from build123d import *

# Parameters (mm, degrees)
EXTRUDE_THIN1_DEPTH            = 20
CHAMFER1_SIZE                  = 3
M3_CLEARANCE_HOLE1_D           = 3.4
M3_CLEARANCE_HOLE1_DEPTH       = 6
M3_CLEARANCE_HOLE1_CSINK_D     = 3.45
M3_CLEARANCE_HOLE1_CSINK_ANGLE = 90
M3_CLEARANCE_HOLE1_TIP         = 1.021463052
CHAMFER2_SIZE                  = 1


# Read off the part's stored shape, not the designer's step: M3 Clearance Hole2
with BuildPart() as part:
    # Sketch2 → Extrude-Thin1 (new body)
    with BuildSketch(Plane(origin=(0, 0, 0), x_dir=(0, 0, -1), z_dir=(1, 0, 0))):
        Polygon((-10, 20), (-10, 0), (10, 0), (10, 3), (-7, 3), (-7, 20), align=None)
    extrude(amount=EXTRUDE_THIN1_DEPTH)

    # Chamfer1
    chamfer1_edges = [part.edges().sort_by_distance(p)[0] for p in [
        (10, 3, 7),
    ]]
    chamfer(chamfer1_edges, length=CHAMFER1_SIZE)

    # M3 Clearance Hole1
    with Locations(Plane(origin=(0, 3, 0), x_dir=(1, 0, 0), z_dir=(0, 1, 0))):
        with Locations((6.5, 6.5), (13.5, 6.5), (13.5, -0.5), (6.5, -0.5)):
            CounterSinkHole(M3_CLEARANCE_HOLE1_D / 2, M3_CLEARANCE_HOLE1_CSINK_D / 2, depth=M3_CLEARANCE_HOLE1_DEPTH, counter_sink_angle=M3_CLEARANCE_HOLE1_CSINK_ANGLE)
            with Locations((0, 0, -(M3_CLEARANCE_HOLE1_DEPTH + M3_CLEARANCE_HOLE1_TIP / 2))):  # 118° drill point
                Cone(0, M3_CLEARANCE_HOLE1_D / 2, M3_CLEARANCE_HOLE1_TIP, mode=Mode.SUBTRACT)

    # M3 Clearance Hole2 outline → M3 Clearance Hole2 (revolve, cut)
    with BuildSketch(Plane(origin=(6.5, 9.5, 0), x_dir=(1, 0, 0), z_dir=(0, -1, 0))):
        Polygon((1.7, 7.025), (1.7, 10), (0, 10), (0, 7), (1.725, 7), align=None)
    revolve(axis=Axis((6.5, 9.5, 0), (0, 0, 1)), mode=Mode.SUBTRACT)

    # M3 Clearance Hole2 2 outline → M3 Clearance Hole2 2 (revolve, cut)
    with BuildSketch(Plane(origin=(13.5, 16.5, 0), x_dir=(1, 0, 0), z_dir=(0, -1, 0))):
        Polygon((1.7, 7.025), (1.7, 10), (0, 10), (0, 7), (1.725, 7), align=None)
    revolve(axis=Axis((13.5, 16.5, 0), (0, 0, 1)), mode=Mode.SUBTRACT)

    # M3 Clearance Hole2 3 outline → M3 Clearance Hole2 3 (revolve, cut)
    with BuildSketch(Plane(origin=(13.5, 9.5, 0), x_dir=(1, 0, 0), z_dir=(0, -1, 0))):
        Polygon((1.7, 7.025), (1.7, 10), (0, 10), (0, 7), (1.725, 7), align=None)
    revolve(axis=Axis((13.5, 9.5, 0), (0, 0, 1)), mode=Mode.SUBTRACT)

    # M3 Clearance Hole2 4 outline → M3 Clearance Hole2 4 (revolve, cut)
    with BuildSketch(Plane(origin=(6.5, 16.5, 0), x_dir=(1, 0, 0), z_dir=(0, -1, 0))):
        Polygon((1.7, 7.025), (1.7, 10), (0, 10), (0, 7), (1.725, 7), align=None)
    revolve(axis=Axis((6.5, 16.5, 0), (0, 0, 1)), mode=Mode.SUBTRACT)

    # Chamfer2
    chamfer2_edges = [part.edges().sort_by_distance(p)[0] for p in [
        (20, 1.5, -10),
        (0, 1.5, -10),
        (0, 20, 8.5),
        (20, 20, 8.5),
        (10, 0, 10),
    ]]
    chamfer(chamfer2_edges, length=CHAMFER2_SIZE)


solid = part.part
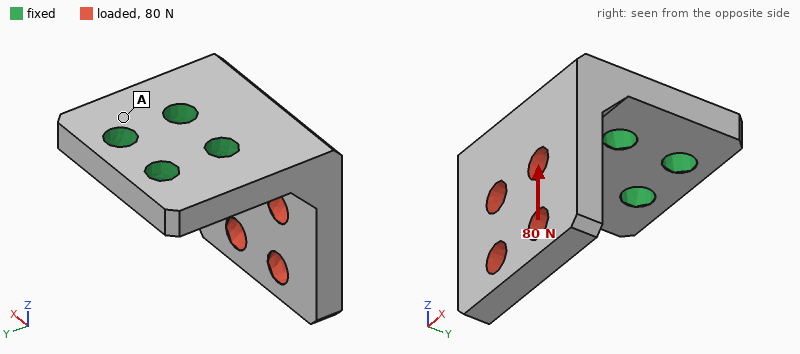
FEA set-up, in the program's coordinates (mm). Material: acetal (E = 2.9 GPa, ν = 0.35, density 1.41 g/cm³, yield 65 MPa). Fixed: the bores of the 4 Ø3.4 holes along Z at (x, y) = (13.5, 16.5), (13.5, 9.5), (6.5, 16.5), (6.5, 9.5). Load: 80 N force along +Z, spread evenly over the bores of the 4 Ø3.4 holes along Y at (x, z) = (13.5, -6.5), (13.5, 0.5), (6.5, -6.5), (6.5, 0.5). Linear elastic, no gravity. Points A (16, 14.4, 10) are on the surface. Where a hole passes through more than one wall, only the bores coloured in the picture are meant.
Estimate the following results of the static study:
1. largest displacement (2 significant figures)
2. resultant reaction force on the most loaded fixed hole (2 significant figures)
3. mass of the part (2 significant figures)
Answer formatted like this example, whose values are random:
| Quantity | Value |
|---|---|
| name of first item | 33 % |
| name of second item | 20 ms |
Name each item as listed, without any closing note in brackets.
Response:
| Quantity | Value |
|---|---|
| largest displacement | 0.27 mm |
| resultant reaction force on the most loaded fixed hole | 46 N |
| mass of the part | 2.9 g |
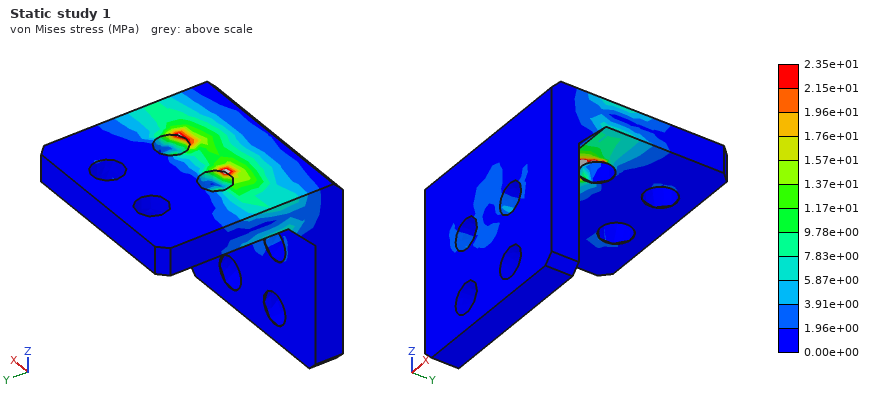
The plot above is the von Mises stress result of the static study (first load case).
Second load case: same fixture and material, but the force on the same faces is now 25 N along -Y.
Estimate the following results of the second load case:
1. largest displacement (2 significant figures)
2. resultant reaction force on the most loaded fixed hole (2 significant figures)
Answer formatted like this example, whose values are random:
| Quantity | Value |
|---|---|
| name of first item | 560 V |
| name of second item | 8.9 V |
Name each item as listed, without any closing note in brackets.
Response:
| Quantity | Value |
|---|---|
| largest displacement | 0.31 mm |
| resultant reaction force on the most loaded fixed hole | 13 N |
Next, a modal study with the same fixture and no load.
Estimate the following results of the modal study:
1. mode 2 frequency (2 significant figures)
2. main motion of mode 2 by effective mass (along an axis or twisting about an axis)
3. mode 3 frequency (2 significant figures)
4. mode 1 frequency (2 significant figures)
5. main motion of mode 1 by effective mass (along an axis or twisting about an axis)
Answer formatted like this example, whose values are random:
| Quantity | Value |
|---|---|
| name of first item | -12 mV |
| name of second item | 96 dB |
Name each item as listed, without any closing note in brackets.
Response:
| Quantity | Value |
|---|---|
| mode 2 frequency | 3000 Hz |
| main motion of mode 2 by effective mass | along X |
| mode 3 frequency | 4600 Hz |
| mode 1 frequency | 1700 Hz |
| main motion of mode 1 by effective mass | along Y |
